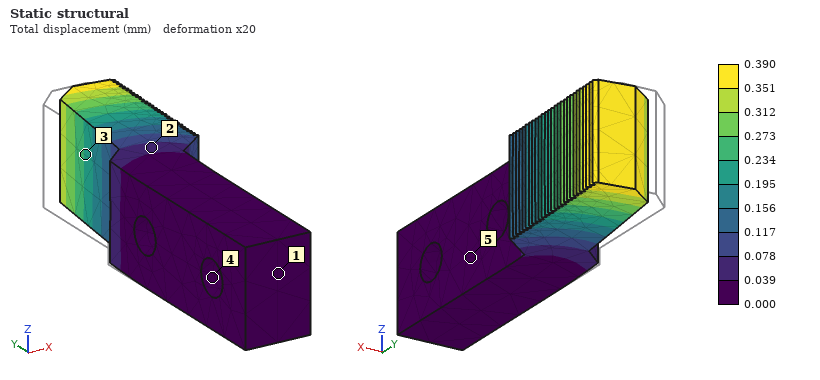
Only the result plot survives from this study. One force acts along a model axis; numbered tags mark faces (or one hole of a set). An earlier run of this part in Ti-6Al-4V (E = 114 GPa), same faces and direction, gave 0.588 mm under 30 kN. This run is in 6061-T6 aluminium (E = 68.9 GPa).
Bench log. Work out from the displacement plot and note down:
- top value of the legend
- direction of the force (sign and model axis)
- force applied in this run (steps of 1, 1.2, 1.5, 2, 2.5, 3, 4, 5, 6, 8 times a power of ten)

0.390 mm
+X
12 kN
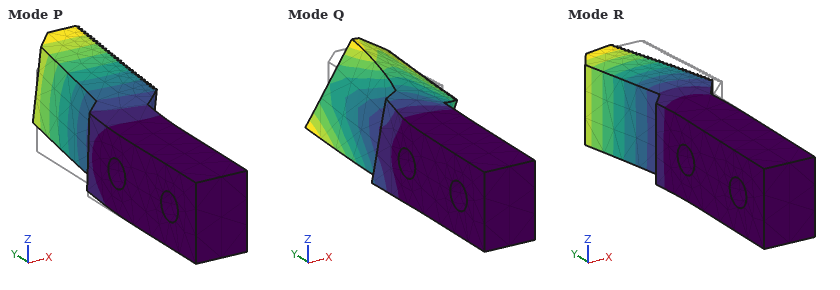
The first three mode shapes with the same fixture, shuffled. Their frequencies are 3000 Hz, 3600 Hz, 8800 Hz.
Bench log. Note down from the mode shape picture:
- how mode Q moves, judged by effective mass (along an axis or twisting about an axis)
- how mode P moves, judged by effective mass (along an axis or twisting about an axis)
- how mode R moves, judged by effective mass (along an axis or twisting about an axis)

twisting about Y
along Z
along X
